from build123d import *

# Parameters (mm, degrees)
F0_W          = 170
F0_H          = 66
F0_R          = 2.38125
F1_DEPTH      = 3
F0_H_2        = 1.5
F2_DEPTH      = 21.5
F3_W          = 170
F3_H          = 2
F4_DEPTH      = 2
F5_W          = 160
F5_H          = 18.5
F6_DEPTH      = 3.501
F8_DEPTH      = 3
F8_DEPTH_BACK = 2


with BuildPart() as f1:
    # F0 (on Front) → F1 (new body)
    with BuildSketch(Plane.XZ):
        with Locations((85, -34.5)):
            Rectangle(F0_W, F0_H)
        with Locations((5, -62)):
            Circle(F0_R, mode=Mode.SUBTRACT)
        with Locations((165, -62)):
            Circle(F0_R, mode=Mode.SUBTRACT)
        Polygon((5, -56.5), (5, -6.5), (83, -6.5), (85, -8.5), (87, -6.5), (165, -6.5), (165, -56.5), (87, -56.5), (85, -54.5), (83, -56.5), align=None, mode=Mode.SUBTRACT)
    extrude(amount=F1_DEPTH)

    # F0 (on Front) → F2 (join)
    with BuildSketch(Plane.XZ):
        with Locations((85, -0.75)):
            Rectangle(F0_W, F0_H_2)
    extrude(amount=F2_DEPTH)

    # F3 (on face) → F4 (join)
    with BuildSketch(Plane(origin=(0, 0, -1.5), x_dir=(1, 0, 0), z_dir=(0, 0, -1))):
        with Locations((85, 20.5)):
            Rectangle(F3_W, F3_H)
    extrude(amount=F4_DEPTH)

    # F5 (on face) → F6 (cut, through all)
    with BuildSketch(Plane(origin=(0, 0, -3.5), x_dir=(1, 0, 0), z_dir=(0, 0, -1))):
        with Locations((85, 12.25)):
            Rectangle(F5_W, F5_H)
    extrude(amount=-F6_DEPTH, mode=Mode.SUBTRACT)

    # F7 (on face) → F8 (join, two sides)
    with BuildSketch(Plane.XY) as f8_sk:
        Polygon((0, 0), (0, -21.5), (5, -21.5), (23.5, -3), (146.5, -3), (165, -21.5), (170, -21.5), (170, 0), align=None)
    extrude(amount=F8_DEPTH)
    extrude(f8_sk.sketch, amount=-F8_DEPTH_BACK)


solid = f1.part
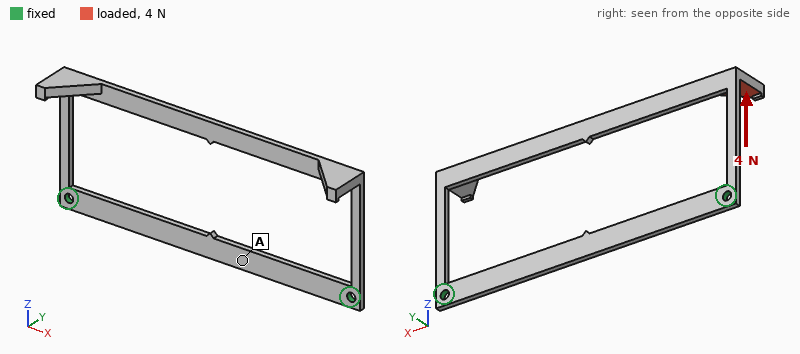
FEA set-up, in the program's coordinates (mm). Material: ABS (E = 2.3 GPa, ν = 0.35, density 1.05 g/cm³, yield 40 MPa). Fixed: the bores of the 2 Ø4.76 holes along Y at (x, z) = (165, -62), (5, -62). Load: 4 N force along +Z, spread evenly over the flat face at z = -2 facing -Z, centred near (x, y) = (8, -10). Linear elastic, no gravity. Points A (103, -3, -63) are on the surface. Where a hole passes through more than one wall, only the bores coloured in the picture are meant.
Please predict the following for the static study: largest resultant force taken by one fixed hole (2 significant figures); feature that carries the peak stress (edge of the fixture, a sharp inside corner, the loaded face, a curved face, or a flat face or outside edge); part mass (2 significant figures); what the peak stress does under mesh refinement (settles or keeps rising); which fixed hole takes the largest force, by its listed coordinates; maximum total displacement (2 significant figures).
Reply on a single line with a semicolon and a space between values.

3.9 N; a sharp inside corner; 15 g; keeps rising; (5, -62); 1.9 mm
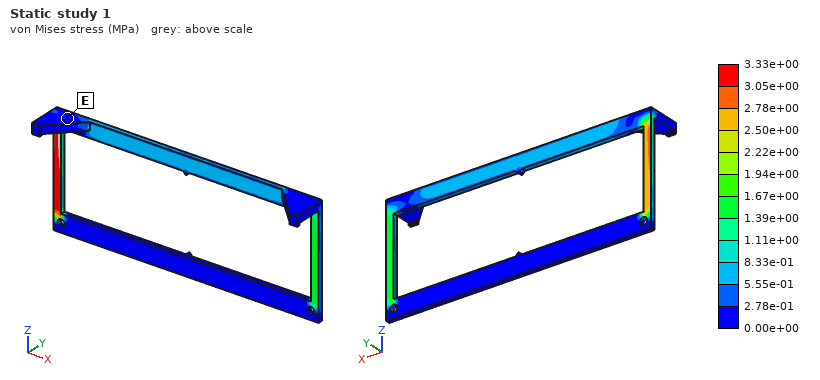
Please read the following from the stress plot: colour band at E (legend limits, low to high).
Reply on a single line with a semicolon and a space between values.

0.00e+00 to 2.78e-01 MPa
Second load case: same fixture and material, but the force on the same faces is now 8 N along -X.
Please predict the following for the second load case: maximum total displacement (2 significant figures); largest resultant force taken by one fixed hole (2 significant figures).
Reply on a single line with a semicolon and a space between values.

1.9 mm; 4.3 N
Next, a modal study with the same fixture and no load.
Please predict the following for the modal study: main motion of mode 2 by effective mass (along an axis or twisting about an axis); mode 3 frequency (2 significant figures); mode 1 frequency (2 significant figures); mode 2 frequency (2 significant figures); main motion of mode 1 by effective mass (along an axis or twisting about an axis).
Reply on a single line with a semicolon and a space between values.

twisting about Z; 140 Hz; 45 Hz; 91 Hz; along Y
